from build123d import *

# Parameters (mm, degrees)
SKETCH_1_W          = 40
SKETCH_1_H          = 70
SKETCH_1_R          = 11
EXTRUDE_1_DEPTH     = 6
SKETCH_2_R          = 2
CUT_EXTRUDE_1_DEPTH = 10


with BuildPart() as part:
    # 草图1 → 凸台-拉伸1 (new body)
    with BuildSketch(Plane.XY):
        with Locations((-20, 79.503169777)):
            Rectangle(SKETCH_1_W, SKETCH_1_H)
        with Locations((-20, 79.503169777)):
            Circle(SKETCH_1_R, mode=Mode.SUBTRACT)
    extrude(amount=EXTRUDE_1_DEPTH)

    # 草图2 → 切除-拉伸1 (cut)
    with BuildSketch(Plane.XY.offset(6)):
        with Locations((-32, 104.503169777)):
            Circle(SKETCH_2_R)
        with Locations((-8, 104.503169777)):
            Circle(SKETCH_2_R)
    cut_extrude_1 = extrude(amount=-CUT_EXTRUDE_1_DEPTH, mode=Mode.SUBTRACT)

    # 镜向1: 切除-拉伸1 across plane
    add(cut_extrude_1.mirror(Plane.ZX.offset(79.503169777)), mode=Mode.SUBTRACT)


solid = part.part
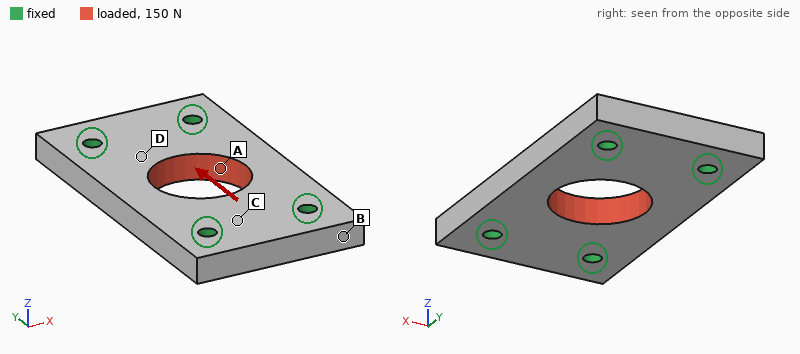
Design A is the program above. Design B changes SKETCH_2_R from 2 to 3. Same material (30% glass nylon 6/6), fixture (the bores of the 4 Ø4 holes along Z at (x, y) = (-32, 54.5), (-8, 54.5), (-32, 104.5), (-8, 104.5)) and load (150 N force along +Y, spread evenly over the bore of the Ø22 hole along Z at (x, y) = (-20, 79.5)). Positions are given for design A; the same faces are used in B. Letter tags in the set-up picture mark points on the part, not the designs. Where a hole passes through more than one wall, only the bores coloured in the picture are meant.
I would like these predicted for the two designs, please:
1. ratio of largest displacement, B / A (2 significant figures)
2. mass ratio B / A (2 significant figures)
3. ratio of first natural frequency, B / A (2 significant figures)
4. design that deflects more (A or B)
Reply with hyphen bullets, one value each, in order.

- 0.91
- 0.97
- 1.1
- A
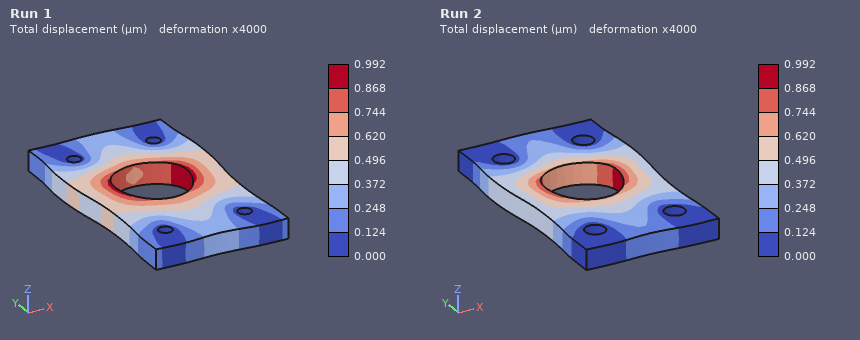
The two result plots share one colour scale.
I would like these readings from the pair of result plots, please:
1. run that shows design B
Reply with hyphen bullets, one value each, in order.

- Run 2
